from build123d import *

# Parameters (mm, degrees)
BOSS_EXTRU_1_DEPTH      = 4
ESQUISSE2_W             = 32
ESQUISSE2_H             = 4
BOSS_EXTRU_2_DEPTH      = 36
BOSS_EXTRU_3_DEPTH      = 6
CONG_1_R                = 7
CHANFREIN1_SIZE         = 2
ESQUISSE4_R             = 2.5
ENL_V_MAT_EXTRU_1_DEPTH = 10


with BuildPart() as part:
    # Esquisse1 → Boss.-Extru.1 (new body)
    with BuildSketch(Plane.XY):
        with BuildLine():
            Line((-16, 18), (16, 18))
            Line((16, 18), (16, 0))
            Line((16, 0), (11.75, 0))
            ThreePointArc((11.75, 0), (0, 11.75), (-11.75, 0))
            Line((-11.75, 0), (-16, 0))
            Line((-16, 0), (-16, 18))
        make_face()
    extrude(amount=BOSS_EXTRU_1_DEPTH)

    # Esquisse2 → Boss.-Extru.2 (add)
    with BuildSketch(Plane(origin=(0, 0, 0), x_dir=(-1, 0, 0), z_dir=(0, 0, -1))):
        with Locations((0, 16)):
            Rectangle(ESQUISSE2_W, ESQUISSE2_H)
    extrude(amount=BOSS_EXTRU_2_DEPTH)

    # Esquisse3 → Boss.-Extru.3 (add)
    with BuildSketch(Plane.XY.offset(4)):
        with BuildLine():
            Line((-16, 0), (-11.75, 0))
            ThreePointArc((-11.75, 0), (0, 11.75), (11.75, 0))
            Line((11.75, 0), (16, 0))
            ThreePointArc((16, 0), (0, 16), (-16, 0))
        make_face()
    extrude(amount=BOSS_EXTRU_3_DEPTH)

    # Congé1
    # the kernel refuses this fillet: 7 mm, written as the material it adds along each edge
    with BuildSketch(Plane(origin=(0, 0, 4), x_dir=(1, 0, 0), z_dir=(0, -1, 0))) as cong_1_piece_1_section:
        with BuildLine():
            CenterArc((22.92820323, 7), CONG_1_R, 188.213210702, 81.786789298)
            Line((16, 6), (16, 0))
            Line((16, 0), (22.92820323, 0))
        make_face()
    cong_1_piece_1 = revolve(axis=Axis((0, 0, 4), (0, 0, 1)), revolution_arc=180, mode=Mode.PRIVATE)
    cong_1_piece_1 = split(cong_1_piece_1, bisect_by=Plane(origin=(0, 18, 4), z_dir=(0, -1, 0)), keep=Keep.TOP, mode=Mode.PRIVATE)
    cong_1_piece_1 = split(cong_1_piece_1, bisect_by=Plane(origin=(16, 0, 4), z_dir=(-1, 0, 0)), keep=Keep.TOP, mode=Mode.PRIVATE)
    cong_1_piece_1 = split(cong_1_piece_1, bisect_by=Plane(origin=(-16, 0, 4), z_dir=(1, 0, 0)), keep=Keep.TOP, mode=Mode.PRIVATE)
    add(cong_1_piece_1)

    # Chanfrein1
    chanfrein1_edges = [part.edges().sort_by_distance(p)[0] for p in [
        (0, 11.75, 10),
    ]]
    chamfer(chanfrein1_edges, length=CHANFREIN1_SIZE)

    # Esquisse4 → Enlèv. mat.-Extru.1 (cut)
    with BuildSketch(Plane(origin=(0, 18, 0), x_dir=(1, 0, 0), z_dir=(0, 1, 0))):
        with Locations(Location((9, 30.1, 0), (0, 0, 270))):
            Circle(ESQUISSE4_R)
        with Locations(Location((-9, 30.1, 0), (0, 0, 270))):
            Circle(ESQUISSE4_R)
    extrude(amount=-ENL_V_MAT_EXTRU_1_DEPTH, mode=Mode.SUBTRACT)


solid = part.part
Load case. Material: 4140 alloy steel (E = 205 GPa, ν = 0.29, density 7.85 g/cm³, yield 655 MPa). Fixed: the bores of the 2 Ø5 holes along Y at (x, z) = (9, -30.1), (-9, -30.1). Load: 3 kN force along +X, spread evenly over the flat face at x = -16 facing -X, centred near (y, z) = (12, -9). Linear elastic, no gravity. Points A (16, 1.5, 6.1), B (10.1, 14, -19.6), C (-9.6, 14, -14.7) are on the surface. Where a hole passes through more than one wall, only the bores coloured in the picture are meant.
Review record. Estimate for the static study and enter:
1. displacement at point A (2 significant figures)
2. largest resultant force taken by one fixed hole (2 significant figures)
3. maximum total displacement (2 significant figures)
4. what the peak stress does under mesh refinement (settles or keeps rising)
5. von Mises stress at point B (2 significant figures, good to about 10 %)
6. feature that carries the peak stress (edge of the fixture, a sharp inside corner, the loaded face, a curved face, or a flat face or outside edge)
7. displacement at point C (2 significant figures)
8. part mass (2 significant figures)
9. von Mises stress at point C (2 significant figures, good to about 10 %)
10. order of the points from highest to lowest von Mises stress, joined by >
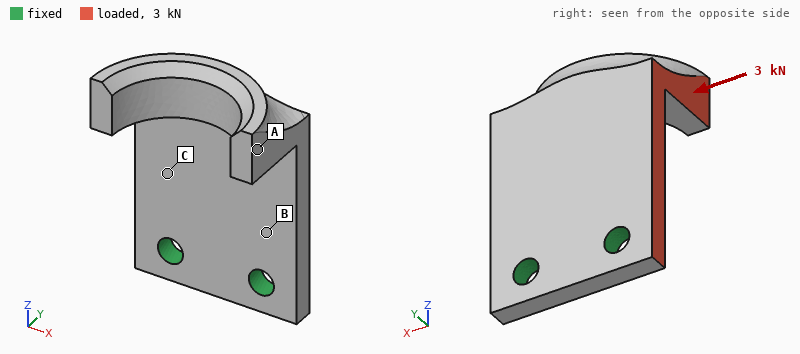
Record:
0.10 mm
3.5 kN
0.14 mm
keeps rising
95 MPa
edge of the fixture
0.021 mm
57 g
130 MPa
C > B > A
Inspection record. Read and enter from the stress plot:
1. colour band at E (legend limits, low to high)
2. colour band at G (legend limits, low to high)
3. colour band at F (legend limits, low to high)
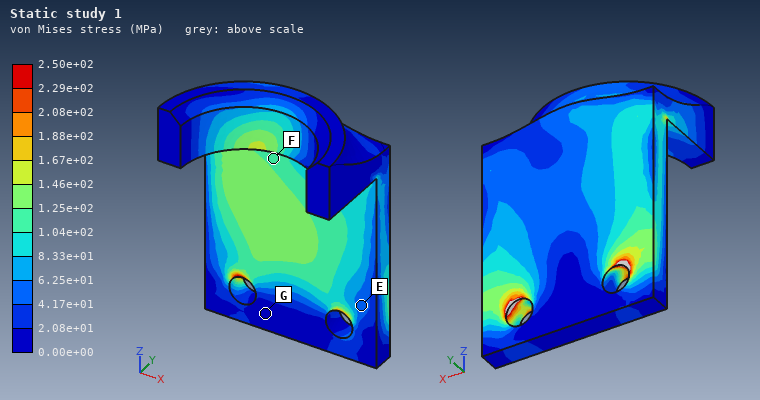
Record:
4.17e+01 to 6.25e+01 MPa
0.00e+00 to 2.08e+01 MPa
1.04e+02 to 1.25e+02 MPa
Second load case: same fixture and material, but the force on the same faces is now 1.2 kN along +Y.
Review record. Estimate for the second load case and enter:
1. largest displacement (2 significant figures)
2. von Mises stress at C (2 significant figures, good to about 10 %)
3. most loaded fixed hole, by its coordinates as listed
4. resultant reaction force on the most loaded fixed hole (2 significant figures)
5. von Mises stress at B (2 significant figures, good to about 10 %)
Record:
0.41 mm
170 MPa
(-9, -30.1)
1.4 kN
170 MPa
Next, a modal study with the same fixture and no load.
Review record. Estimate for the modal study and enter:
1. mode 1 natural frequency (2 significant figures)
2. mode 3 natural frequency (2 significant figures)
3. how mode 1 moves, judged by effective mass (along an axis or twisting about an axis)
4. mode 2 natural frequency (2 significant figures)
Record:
1600 Hz
8200 Hz
along Y
3800 Hz
